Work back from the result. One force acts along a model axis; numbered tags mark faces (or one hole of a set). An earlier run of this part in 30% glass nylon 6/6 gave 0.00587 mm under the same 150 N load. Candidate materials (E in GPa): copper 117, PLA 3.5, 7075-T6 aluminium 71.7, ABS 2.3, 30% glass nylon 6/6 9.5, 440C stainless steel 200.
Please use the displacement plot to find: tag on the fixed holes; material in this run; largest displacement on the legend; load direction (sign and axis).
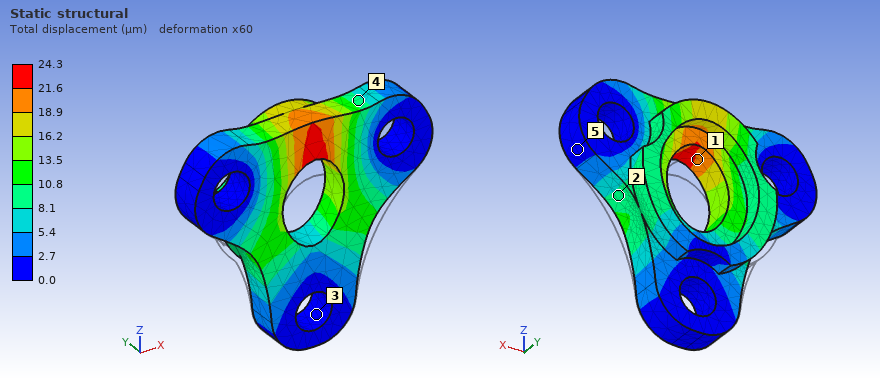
3
ABS
24.3 µm
+Z
